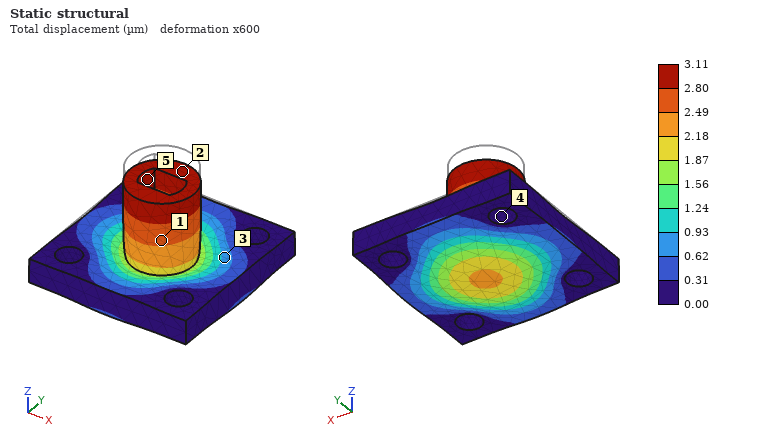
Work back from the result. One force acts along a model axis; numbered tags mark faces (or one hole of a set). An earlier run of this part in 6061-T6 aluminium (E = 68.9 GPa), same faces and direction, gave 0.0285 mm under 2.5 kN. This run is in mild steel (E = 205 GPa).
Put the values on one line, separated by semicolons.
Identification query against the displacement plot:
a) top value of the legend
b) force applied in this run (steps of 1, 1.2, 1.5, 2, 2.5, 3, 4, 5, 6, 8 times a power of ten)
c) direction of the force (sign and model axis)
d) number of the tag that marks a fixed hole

3.11 µm; 800 N; -Z; 4
